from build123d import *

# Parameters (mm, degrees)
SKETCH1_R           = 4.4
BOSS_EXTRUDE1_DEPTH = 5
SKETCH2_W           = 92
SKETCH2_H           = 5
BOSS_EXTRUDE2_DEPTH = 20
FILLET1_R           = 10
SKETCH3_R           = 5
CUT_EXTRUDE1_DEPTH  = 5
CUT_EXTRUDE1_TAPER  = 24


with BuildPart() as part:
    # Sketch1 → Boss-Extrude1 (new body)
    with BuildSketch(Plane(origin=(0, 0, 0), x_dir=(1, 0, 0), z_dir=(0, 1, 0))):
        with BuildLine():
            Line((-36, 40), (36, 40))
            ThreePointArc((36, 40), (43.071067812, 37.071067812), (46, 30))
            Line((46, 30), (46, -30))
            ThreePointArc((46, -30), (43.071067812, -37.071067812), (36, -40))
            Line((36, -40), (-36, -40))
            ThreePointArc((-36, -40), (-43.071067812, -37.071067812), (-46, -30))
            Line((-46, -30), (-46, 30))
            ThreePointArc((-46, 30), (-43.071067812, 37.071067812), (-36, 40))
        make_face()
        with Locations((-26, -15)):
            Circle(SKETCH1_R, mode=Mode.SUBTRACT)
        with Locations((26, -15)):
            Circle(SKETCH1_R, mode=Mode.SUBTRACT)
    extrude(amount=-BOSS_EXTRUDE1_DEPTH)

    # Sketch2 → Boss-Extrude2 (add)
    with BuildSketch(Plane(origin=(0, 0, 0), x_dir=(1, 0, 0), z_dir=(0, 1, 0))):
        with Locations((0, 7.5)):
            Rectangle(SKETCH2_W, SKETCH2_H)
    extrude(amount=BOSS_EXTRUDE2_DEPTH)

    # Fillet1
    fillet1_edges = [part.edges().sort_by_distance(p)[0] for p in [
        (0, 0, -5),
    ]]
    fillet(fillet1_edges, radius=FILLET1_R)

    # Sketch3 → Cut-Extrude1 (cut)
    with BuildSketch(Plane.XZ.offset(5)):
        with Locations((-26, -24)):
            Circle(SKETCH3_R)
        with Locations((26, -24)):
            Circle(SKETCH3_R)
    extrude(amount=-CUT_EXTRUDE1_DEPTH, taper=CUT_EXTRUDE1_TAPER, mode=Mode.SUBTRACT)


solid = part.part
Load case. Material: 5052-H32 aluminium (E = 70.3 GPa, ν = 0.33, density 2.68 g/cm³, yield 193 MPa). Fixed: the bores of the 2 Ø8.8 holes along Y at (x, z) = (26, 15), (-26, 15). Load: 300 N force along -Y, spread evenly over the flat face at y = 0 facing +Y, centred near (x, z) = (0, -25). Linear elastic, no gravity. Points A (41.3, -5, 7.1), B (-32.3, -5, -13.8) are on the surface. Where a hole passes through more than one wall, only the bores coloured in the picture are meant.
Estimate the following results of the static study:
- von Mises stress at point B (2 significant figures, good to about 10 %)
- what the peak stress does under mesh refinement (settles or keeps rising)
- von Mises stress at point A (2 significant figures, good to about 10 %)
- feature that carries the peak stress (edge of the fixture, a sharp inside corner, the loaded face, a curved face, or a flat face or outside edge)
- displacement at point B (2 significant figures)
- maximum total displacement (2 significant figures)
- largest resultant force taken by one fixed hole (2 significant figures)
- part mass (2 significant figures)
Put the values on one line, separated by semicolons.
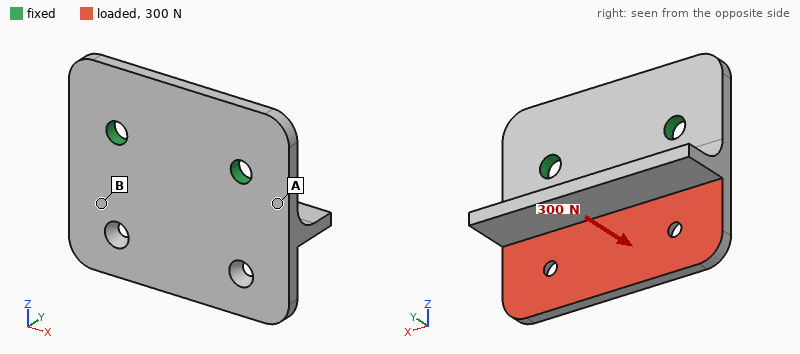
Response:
7.4 MPa; keeps rising; 19 MPa; edge of the fixture; 0.045 mm; 0.12 mm; 150 N; 120 g
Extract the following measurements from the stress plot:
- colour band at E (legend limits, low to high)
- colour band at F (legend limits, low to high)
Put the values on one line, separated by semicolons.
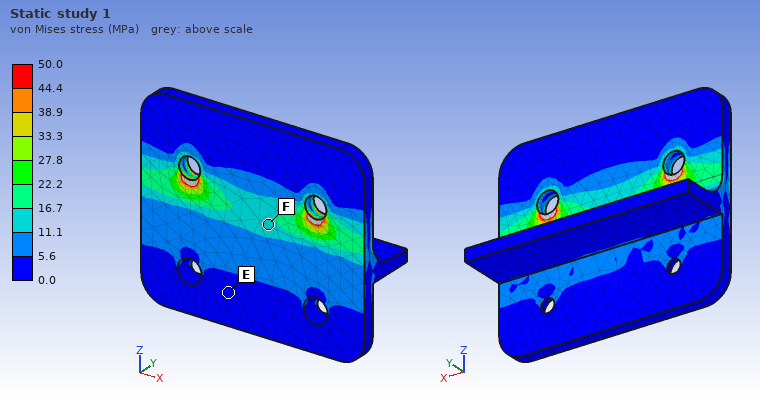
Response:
0.0 to 5.6 MPa; 11.1 to 16.7 MPa
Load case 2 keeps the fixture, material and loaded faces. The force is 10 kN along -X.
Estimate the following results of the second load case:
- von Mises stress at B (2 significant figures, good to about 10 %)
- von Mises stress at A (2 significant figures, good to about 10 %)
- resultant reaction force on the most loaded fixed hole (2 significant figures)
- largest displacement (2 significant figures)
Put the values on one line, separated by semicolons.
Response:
22 MPa; 34 MPa; 8.5 kN; 0.14 mm
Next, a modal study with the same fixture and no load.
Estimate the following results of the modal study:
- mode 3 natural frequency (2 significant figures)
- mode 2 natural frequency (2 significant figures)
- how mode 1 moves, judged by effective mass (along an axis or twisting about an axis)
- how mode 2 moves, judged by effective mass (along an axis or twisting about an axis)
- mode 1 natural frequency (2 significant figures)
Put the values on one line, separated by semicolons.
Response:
6300 Hz; 2700 Hz; along Y; twisting about Z; 1400 Hz
